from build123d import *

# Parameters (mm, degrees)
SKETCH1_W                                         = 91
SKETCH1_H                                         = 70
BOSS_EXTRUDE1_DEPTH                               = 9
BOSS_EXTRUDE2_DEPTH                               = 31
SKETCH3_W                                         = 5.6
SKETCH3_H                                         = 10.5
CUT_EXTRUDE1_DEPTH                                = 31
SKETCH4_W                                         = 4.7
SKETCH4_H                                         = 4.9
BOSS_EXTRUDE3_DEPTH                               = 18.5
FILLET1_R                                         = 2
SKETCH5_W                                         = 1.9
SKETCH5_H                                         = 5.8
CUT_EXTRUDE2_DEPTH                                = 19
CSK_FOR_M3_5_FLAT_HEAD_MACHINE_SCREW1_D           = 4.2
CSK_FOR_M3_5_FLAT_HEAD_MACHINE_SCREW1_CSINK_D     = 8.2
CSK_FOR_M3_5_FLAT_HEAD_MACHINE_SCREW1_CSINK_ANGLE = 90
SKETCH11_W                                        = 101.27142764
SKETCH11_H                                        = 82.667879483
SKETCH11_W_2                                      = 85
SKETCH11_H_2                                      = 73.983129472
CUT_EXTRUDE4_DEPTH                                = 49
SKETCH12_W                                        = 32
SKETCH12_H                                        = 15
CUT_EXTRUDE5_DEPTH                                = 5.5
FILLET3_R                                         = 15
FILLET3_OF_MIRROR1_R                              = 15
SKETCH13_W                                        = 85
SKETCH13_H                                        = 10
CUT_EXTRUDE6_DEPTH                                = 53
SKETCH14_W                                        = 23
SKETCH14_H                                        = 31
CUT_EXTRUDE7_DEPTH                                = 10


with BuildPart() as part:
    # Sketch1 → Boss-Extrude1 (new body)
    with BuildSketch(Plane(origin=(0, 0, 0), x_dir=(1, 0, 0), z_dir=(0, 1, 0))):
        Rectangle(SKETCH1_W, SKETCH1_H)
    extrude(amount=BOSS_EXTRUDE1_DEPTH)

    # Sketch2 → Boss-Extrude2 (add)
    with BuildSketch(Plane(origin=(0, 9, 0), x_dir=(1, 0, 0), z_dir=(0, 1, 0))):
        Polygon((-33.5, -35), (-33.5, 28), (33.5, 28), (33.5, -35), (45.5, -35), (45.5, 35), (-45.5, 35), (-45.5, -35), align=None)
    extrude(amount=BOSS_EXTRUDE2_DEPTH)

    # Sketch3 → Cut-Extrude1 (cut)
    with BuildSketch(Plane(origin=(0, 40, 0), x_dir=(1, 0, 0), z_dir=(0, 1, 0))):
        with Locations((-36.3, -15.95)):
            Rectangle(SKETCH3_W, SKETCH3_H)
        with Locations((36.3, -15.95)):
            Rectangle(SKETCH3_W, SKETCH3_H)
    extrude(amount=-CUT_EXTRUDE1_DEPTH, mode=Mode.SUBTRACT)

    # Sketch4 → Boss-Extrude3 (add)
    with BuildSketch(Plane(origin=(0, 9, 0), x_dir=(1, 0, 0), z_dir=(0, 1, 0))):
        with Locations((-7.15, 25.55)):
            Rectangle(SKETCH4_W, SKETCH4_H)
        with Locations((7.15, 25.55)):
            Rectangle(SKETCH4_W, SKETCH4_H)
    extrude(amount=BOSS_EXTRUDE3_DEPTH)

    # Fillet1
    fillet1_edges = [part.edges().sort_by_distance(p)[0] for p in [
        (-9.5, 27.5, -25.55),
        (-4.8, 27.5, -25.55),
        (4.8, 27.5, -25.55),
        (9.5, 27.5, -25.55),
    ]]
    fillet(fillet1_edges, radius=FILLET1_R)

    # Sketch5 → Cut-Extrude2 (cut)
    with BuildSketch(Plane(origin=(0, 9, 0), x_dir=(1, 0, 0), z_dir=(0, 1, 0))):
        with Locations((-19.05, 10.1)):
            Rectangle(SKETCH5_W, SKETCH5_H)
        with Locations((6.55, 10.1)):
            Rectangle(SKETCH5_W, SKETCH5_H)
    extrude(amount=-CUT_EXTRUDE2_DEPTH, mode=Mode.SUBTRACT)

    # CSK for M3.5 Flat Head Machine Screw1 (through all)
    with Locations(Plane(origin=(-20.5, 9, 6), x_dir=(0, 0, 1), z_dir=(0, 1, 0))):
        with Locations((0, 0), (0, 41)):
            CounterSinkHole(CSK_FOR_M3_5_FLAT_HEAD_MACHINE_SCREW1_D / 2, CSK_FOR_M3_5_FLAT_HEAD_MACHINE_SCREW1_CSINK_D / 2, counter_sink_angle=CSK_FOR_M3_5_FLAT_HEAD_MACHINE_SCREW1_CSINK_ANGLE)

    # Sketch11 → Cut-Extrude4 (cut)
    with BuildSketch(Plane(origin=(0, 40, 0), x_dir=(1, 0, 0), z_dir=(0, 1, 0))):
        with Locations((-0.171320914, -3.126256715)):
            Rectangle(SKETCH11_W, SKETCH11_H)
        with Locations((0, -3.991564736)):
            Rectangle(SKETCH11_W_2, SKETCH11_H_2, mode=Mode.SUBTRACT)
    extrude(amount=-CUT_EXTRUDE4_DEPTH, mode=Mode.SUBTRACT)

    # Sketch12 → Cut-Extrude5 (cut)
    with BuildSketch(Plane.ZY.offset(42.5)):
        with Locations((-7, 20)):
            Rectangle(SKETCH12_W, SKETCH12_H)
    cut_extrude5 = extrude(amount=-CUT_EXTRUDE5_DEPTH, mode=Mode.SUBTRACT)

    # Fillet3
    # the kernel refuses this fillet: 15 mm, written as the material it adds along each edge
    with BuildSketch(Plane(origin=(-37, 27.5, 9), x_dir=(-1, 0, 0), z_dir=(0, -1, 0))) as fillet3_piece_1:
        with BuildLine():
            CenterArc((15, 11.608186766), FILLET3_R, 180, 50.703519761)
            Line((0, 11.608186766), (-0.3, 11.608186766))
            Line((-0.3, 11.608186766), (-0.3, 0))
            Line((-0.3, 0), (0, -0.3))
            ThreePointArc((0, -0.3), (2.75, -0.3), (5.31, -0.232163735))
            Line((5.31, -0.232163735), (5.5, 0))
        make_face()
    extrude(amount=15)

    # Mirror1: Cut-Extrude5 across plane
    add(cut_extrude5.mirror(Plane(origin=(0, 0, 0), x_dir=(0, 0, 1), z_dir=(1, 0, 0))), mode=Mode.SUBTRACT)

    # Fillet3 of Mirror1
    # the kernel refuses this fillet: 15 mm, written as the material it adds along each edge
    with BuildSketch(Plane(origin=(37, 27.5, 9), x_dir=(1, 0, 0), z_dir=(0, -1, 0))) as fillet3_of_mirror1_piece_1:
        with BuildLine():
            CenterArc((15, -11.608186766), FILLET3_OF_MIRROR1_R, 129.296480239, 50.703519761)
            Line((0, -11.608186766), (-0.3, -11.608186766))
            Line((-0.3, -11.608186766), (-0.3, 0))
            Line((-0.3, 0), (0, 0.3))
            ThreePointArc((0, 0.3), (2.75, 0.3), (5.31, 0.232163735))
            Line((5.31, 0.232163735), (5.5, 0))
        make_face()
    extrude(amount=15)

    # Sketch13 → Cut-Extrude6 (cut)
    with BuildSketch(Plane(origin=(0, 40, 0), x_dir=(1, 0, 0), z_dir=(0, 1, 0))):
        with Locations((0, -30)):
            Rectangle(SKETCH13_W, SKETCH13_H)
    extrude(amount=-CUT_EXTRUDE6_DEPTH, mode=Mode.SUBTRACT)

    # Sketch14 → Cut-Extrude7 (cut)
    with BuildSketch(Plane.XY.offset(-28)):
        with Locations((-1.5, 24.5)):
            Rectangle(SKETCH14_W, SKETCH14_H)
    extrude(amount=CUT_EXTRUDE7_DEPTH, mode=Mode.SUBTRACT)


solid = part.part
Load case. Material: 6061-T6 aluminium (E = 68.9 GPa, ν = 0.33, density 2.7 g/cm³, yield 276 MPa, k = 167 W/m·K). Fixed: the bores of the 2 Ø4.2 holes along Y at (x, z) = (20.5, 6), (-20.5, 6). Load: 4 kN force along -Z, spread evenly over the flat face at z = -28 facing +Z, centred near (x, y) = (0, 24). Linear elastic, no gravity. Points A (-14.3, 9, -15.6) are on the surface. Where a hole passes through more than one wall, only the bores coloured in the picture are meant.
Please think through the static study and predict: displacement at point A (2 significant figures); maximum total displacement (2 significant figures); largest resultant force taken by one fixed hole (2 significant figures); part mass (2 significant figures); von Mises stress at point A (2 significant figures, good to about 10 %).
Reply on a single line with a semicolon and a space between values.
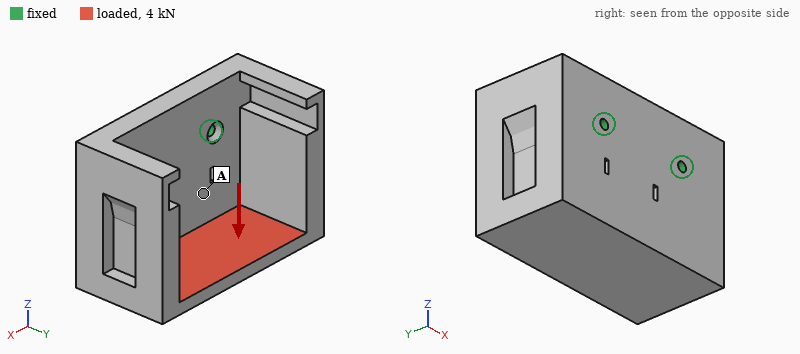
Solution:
0.083 mm; 0.37 mm; 2.0 kN; 210 g; 29 MPa
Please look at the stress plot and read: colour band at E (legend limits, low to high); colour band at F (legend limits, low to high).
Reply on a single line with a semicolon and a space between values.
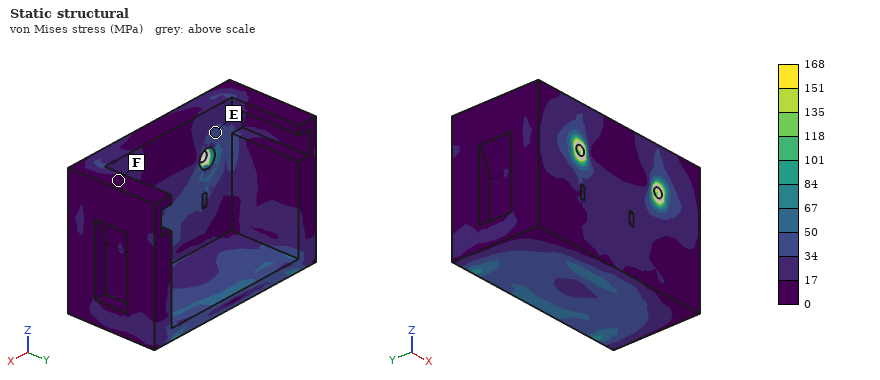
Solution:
34 to 50 MPa; 0 to 17 MPa
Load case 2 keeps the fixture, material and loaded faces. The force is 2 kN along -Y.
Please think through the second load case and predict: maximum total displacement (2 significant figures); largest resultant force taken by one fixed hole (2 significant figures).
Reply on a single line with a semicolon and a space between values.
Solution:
0.18 mm; 1.0 kN
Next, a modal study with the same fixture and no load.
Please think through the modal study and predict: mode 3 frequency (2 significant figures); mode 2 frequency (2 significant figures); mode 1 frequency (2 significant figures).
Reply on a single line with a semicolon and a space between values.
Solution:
4200 Hz; 2300 Hz; 1800 Hz
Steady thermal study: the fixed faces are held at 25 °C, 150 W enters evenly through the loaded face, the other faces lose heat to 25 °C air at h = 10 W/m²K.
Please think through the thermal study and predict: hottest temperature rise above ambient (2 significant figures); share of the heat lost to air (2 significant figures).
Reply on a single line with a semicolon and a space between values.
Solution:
74 K; 4.9 %
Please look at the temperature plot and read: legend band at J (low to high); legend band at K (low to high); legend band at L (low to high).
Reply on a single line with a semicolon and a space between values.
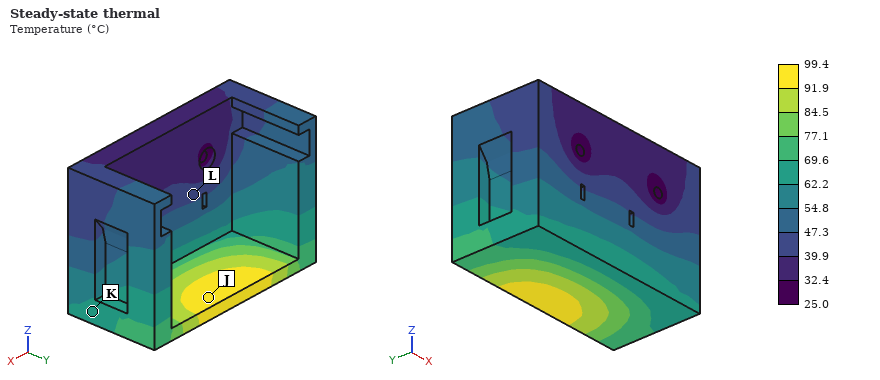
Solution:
91.9 to 99.4 °C; 62.2 to 69.6 °C; 39.9 to 47.3 °C
